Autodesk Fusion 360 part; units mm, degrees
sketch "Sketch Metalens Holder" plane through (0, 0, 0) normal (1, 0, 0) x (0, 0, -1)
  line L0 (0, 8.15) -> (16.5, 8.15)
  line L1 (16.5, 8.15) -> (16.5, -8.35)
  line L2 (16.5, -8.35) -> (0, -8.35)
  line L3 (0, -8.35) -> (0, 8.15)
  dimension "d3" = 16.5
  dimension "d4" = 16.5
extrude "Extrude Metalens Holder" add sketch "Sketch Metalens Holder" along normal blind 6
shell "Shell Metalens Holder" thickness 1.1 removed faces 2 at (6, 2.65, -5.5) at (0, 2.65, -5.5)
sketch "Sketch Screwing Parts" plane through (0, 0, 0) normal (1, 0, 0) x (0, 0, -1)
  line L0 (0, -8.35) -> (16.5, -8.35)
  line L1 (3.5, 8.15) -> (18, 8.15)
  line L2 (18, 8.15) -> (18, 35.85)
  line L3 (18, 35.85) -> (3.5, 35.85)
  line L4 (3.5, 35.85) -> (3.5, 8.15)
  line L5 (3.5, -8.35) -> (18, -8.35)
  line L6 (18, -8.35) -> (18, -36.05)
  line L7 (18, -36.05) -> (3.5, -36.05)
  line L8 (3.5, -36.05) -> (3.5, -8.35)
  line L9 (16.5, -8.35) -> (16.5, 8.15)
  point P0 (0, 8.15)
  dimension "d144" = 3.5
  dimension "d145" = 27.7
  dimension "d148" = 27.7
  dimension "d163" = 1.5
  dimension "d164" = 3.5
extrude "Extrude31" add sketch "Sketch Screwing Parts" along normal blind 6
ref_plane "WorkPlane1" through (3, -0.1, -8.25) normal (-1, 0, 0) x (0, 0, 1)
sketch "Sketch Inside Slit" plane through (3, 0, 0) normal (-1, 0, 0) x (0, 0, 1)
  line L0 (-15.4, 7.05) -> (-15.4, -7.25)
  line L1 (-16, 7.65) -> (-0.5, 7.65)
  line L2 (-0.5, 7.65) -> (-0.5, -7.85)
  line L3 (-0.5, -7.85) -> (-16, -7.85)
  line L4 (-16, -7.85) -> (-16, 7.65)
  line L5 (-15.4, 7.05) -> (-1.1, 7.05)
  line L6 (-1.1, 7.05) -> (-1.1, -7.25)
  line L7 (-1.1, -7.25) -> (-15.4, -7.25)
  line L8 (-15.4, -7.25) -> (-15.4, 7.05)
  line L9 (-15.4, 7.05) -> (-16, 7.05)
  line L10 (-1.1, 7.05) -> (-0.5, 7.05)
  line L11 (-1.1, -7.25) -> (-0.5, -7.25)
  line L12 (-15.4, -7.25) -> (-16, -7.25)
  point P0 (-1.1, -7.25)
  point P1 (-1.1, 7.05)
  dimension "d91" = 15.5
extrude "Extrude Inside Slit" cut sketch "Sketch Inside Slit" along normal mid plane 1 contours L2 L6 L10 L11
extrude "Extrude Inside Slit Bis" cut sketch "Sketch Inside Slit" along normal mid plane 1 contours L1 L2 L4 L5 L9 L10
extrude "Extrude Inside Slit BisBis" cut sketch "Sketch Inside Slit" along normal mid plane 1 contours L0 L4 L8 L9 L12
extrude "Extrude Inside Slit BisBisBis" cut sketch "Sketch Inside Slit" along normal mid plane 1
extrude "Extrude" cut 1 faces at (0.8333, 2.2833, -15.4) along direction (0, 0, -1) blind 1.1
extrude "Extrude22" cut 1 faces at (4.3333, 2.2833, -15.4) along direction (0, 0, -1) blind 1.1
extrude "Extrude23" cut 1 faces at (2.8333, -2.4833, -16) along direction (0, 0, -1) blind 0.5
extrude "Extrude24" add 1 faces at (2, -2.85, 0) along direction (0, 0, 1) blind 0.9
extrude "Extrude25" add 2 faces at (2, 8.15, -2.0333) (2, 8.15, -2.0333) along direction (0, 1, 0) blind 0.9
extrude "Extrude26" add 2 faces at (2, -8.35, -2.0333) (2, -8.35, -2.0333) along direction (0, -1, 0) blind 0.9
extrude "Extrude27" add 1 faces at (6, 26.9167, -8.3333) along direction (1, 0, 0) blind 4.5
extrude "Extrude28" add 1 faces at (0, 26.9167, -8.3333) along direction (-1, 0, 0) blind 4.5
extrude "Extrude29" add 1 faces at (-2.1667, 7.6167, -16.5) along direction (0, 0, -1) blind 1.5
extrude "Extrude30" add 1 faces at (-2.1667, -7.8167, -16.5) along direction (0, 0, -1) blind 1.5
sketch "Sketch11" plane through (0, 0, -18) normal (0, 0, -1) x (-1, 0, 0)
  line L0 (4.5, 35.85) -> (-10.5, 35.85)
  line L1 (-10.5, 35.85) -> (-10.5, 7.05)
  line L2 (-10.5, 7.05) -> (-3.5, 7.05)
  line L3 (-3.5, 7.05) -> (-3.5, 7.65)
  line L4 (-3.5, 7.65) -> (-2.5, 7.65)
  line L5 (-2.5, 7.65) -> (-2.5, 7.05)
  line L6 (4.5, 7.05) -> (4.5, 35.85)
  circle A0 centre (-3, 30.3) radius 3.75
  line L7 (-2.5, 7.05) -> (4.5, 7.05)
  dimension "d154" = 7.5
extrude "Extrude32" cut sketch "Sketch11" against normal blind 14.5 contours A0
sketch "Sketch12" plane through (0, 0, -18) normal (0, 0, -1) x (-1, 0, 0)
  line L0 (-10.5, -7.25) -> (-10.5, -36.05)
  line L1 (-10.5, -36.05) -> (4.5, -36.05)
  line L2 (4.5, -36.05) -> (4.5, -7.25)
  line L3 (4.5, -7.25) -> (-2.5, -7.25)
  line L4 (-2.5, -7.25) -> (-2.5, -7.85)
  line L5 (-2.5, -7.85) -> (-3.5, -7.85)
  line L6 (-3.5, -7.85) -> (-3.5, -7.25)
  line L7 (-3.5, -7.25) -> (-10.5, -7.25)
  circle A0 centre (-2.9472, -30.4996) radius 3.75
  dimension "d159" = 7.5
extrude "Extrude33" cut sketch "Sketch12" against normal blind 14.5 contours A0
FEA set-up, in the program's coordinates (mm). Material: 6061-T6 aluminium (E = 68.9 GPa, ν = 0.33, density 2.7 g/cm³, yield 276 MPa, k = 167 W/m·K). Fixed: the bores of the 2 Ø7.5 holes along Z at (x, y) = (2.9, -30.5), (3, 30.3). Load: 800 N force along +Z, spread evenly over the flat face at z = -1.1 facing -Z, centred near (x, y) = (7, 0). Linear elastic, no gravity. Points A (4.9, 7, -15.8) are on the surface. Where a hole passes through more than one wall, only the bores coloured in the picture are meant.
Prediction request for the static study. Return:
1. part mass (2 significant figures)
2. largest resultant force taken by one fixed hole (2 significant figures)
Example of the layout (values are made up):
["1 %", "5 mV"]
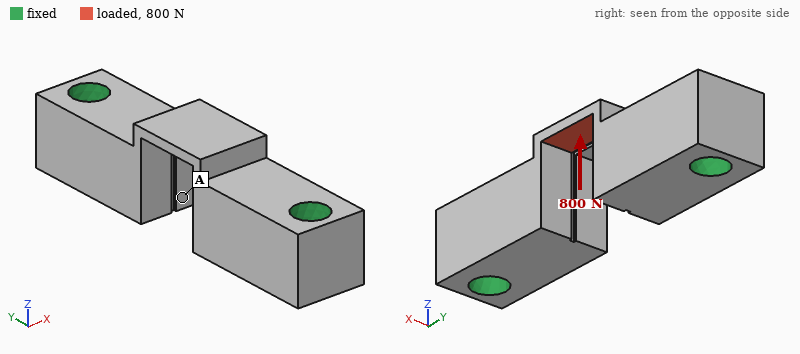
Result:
["32 g", "540 N"]
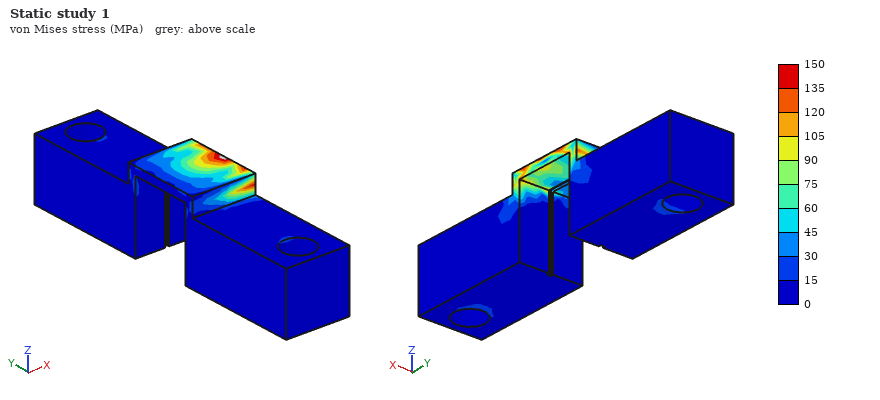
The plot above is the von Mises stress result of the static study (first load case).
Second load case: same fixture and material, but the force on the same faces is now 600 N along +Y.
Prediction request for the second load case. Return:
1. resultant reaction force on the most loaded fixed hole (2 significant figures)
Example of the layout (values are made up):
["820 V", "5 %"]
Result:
["310 N"]
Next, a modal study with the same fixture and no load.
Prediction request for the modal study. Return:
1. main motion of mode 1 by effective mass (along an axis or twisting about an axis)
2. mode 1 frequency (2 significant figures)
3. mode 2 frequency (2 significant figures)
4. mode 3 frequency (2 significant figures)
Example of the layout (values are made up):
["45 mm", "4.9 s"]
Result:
["along X", "16 kHz", "19 kHz", "19 kHz"]
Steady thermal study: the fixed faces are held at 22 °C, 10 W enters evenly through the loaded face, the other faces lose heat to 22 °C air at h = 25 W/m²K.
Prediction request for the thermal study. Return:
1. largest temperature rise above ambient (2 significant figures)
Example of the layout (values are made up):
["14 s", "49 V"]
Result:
["15 K"]
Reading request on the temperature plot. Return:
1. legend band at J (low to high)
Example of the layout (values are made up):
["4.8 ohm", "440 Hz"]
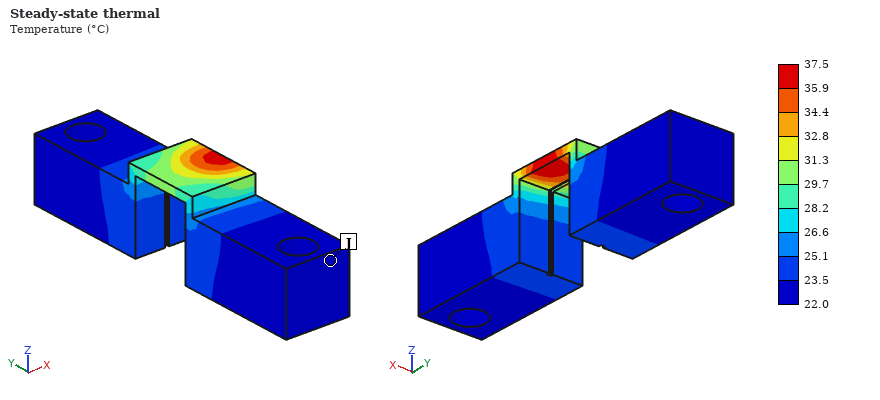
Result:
["22.0 to 23.5 °C"]
